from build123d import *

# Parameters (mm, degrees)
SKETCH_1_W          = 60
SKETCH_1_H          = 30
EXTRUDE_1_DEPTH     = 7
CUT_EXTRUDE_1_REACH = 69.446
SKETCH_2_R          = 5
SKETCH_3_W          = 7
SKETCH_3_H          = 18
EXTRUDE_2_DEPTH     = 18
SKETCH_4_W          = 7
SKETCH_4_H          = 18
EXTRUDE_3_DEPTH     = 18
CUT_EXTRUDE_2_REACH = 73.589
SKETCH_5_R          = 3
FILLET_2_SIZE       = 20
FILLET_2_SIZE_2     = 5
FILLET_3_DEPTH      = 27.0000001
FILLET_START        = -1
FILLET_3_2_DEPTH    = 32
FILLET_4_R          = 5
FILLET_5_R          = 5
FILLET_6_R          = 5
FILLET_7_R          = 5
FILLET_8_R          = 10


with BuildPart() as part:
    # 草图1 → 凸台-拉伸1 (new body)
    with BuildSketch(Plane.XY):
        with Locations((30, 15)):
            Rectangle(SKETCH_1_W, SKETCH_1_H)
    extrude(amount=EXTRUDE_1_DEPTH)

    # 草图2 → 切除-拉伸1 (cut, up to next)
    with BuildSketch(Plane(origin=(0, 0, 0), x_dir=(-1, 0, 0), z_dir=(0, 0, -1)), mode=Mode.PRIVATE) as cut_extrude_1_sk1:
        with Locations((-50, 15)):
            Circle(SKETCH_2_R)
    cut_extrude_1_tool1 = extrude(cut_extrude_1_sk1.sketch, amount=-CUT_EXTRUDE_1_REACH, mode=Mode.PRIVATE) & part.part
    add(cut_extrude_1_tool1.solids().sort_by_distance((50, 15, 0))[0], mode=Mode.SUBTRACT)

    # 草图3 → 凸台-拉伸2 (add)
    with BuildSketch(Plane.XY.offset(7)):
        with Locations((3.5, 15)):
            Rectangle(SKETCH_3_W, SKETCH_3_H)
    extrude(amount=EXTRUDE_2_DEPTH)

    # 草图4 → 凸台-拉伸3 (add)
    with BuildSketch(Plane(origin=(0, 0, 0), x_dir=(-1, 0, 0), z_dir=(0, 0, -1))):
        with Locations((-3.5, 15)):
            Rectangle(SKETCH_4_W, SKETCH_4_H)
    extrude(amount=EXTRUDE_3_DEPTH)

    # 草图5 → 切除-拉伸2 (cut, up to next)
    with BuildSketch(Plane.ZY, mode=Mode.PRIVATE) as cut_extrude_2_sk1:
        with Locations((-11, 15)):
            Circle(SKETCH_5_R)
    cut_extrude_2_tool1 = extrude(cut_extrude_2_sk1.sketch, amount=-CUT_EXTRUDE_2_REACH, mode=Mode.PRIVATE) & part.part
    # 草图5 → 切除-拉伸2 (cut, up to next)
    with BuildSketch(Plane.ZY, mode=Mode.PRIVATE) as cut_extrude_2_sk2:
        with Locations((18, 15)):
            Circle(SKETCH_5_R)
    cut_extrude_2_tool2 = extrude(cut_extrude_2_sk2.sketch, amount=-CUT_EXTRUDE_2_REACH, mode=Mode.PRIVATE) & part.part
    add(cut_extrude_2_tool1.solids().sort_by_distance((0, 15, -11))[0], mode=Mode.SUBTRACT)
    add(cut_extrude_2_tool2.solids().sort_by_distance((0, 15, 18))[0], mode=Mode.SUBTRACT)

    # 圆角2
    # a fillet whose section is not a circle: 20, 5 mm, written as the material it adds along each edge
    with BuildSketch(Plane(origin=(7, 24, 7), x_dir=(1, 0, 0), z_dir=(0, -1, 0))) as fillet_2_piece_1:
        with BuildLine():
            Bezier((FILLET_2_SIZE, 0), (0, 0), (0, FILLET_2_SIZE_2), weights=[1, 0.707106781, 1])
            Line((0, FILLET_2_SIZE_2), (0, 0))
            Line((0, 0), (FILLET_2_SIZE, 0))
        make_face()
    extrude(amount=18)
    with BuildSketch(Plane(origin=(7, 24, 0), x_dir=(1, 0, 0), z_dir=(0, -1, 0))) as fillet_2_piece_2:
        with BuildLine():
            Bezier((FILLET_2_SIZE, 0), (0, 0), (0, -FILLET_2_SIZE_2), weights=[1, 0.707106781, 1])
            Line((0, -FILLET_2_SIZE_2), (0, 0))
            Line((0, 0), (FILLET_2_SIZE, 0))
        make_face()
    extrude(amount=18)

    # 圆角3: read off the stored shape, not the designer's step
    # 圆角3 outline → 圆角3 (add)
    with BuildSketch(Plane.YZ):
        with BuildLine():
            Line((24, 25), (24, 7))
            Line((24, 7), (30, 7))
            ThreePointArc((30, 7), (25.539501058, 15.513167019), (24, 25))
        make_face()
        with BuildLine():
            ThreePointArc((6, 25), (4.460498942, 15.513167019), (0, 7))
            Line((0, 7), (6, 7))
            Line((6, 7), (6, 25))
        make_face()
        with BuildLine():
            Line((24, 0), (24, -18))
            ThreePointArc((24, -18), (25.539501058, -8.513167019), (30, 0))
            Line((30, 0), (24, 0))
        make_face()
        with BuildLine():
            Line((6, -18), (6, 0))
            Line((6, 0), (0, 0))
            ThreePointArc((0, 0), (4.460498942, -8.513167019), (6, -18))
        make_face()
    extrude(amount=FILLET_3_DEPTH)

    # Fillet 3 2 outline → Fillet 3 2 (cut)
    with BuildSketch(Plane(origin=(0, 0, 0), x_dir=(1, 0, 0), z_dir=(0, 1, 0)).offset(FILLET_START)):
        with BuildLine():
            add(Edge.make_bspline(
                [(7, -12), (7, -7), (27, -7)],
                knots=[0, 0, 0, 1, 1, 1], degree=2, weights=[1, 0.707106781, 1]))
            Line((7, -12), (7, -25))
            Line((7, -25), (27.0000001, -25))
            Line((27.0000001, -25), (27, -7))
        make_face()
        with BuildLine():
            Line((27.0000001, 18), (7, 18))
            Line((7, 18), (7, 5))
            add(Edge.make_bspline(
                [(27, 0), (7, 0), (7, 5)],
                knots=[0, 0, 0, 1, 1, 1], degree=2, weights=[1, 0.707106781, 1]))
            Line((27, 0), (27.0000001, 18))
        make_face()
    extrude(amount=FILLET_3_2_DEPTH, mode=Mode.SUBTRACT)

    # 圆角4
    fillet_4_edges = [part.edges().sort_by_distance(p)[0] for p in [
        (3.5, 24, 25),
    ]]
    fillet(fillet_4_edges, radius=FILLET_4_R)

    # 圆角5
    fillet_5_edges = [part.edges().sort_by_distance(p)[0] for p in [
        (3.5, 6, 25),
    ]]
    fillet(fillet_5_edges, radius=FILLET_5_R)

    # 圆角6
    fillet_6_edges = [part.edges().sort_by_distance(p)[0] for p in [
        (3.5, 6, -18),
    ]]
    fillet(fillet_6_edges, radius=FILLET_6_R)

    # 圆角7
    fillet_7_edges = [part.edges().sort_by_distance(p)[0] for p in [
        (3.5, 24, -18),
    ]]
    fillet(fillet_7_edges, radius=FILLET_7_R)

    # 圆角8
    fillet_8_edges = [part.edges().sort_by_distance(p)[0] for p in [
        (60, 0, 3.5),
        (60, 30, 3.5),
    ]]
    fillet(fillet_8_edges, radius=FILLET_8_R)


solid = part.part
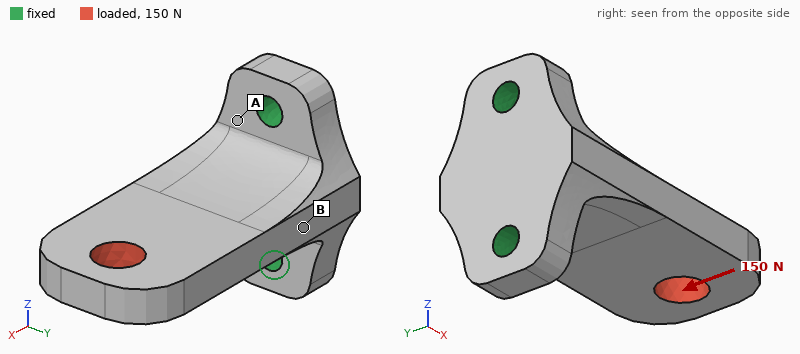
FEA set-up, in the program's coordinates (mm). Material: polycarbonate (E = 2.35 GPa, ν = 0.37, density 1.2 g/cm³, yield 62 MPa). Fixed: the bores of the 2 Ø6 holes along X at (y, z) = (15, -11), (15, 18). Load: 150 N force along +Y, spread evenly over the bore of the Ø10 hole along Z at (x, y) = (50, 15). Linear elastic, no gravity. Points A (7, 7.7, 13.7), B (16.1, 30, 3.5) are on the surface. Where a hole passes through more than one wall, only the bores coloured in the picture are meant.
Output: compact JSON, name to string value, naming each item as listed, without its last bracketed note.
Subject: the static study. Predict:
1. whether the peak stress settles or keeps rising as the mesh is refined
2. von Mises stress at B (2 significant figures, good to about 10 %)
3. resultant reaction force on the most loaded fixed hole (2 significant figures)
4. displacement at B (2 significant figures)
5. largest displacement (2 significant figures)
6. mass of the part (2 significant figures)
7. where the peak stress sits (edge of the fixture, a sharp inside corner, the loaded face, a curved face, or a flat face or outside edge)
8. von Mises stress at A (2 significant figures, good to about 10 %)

{"whether the peak stress settles or keeps rising as the mesh is refined": "keeps rising", "von Mises stress at B": "3.8 MPa", "resultant reaction force on the most loaded fixed hole": "75 N", "displacement at B": "0.28 mm", "largest displacement": "0.90 mm", "mass of the part": "22 g", "where the peak stress sits": "edge of the fixture", "von Mises stress at A": "10 MPa"}
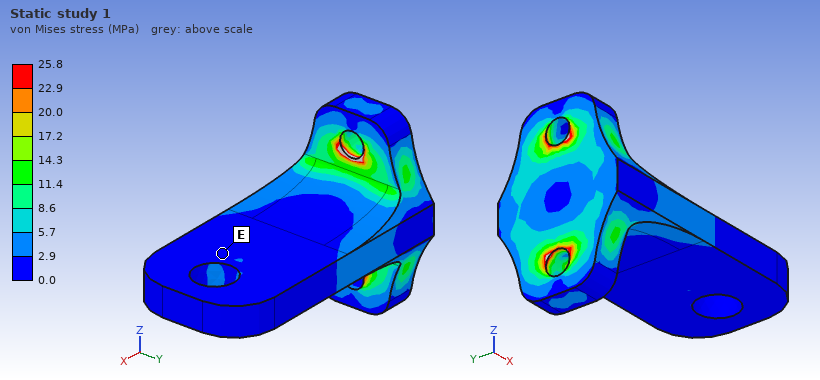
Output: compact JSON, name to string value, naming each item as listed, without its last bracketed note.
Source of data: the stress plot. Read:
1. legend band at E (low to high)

{"legend band at E": "0.0 to 2.9 MPa"}
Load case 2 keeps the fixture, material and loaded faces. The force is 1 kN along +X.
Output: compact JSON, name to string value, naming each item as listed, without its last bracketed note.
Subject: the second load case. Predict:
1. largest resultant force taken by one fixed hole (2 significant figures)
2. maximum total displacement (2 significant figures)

{"largest resultant force taken by one fixed hole": "530 N", "maximum total displacement": "0.21 mm"}
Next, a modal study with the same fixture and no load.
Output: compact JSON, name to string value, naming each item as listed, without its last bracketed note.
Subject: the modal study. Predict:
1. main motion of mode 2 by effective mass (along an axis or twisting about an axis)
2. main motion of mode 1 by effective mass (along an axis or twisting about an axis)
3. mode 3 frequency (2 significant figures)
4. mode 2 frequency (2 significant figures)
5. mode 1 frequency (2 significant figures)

{"main motion of mode 2 by effective mass": "along Y", "main motion of mode 1 by effective mass": "along Z", "mode 3 frequency": "2200 Hz", "mode 2 frequency": "910 Hz", "mode 1 frequency": "780 Hz"}
